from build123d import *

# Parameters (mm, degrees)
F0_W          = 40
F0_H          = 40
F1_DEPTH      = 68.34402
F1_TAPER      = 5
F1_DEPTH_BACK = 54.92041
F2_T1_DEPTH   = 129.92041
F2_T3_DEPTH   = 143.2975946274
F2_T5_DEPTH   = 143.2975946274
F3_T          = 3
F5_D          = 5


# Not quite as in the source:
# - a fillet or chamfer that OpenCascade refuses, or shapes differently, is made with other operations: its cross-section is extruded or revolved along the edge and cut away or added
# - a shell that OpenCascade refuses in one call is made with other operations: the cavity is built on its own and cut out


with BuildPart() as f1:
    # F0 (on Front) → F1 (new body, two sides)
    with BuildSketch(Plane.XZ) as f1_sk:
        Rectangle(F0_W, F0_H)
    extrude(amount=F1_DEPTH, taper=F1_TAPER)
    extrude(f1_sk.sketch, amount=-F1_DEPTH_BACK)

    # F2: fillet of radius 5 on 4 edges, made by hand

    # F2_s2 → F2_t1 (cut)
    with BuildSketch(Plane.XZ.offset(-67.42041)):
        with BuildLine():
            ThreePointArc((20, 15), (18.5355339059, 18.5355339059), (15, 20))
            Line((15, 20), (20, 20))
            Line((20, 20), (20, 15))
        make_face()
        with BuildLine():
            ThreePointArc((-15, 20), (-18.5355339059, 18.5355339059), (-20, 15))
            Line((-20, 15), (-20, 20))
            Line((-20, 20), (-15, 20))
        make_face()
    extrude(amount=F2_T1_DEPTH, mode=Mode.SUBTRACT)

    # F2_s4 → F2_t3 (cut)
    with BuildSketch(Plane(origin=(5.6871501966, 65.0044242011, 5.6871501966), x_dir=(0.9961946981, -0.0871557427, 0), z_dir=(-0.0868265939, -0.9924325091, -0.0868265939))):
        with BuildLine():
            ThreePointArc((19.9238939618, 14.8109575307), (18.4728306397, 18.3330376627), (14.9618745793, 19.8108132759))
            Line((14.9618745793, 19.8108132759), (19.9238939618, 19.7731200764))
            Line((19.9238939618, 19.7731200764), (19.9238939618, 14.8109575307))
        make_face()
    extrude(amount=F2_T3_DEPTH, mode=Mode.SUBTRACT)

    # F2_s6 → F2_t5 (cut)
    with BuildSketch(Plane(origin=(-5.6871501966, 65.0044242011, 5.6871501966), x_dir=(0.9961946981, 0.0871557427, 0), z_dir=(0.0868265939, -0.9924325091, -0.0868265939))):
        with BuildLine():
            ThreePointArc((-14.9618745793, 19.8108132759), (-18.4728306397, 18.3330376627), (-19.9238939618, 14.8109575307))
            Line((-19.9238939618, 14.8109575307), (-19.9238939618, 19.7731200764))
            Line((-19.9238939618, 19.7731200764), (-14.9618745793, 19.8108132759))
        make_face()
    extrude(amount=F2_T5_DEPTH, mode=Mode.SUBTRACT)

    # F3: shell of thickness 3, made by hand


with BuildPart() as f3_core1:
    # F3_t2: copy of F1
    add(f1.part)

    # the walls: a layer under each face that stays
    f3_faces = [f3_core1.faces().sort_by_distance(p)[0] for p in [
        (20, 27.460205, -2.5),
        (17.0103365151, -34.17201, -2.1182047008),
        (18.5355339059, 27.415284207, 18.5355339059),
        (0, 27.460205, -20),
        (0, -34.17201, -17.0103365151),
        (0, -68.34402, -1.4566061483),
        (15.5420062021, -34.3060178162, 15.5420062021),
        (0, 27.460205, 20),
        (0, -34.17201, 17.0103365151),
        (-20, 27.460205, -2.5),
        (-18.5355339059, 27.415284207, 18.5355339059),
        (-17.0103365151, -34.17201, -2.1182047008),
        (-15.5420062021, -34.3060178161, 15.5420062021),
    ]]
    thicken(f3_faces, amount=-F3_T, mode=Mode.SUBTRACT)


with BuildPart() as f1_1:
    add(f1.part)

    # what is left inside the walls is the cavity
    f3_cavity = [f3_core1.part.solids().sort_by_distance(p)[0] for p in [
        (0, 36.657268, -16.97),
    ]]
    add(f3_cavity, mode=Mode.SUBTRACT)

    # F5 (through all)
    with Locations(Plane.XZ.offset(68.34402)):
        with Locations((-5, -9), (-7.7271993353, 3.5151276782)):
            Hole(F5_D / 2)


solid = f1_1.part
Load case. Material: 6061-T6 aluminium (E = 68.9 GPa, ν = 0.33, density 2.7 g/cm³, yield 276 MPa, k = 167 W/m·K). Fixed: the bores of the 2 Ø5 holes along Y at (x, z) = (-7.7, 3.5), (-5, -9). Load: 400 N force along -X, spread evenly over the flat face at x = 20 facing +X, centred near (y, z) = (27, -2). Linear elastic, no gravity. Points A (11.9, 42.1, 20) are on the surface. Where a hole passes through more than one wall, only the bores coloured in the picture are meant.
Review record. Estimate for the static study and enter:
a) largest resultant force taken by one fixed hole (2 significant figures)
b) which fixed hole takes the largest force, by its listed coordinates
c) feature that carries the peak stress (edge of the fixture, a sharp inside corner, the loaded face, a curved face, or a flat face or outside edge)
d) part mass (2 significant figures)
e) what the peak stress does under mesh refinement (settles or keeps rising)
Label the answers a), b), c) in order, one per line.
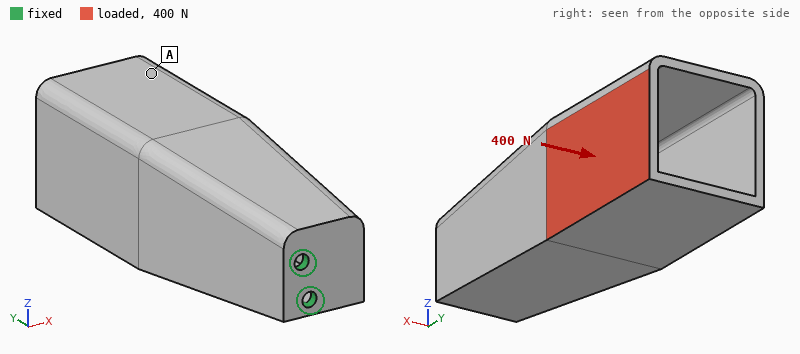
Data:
a) 560 N
b) (-7.7, 3.5)
c) edge of the fixture
d) 140 g
e) keeps rising
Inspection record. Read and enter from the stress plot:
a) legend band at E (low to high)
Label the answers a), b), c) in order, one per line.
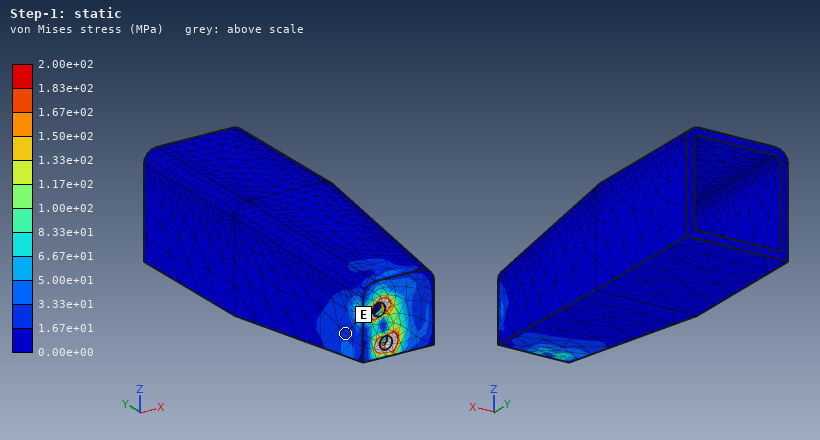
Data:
a) 1.67e+01 to 3.33e+01 MPa
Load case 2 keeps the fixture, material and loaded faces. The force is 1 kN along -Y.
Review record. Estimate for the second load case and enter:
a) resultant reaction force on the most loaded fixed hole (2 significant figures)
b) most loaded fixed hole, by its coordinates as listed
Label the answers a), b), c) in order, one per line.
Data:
a) 790 N
b) (-5, -9)
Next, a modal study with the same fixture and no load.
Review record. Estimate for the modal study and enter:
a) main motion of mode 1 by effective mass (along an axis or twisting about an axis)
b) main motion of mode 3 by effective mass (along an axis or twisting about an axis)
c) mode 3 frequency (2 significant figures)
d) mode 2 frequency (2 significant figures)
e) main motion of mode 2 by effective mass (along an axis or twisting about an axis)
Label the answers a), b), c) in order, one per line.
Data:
a) along X
b) twisting about Y
c) 3200 Hz
d) 780 Hz
e) along Z
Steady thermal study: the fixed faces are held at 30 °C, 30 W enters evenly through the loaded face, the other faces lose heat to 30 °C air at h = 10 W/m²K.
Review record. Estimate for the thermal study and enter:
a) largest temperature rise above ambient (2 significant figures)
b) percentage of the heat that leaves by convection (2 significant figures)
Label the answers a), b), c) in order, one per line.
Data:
a) 48 K
b) 28 %
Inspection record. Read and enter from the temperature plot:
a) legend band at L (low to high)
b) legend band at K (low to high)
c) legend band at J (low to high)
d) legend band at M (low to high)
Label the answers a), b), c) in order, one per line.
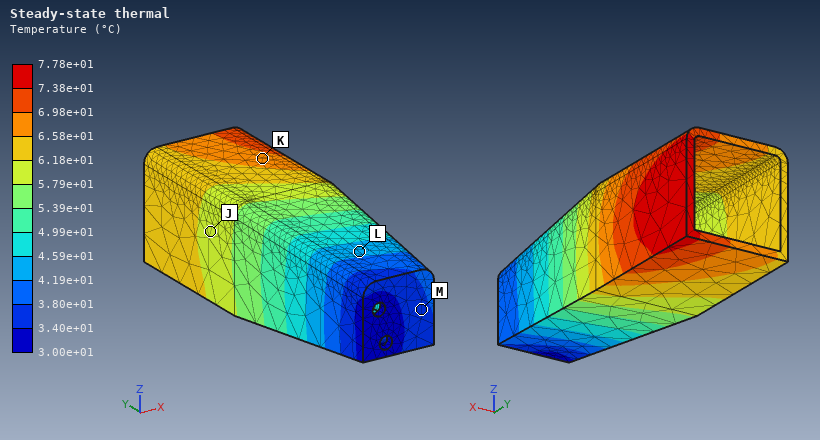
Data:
a) 4.19e+01 to 4.59e+01 °C
b) 6.58e+01 to 6.98e+01 °C
c) 5.79e+01 to 6.18e+01 °C
d) 3.40e+01 to 3.80e+01 °C
